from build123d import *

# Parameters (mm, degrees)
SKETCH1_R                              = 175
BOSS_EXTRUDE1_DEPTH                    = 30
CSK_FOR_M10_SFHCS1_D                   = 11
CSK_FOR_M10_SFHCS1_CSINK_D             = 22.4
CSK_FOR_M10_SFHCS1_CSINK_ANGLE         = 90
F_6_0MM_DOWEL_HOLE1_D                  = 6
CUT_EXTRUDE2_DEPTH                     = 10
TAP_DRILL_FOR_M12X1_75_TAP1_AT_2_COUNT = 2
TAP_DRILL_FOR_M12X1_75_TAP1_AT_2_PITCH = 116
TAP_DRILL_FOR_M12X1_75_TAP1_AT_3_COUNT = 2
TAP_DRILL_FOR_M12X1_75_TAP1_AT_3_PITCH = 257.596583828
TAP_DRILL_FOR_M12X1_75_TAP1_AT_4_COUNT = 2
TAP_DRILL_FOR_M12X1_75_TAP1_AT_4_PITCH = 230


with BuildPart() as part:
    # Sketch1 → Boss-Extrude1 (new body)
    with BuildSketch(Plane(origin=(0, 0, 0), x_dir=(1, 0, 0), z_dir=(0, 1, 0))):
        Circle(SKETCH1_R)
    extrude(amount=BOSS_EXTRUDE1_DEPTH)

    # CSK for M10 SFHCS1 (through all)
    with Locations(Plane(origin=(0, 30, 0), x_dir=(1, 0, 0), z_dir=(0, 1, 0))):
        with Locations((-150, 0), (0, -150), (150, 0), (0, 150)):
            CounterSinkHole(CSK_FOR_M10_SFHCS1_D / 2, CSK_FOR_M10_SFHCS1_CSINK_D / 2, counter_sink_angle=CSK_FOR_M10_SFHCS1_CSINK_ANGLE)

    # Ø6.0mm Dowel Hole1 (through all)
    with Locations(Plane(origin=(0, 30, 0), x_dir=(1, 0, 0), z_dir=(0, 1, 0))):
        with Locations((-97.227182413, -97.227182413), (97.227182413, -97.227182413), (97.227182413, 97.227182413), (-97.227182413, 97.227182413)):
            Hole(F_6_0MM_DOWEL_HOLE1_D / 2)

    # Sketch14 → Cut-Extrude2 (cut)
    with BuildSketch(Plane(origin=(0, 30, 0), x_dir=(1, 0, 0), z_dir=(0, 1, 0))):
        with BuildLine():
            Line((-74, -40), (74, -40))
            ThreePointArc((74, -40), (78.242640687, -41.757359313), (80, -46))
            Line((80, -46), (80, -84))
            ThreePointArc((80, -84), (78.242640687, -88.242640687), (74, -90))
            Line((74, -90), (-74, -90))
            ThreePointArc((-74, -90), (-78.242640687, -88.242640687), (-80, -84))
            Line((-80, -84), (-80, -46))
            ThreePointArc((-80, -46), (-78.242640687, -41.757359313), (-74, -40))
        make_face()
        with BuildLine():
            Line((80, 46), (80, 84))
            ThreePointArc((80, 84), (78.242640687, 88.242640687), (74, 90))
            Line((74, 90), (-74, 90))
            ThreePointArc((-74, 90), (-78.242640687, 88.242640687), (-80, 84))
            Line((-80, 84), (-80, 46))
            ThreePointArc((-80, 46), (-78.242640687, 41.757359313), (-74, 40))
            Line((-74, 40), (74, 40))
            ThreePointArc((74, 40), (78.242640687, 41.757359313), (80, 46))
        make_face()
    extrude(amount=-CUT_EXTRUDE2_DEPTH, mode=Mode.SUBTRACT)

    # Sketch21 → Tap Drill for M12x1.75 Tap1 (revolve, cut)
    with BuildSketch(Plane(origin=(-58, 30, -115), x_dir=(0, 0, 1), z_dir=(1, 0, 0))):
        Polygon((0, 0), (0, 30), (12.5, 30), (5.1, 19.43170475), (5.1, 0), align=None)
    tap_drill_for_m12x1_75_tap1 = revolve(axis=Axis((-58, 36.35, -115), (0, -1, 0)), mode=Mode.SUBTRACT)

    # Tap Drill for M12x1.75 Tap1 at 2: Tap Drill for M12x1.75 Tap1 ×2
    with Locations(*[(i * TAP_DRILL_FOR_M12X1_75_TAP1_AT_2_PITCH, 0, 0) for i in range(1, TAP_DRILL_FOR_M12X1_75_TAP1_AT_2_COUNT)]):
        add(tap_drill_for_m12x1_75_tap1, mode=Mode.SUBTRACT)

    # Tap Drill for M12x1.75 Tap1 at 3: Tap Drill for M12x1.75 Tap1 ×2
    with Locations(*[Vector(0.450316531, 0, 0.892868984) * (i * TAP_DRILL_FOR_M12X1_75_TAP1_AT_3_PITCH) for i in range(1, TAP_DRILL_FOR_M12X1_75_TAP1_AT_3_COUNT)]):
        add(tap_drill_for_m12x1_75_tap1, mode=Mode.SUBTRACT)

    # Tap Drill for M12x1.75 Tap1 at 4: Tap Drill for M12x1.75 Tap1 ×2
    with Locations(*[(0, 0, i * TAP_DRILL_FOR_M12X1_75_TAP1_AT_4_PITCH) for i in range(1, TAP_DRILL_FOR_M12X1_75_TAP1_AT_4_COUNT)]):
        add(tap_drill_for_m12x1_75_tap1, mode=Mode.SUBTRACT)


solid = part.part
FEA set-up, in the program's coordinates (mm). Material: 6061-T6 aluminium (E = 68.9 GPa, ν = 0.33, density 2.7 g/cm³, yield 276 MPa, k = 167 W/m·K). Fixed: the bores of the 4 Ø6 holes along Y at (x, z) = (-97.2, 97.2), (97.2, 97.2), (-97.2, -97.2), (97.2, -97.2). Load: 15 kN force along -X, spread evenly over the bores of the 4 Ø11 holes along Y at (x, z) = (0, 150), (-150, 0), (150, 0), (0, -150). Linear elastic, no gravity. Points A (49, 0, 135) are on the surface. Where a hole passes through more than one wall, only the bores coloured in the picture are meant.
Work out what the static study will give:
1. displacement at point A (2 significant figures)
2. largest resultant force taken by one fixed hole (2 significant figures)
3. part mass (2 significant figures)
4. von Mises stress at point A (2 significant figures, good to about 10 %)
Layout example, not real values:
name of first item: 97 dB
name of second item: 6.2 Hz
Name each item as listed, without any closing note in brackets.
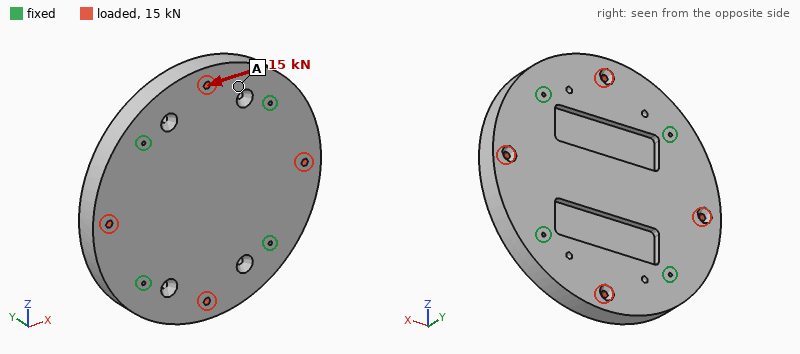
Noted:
displacement at point A: 2.1 µm
largest resultant force taken by one fixed hole: 3.9 kN
part mass: 7.3 kg
von Mises stress at point A: 1.6 MPa
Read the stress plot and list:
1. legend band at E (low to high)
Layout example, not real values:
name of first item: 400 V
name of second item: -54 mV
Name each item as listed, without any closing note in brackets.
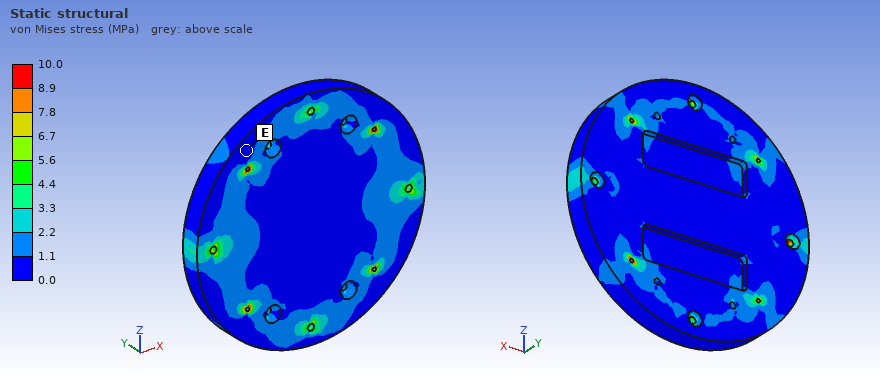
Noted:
legend band at E: 0.0 to 1.1 MPa
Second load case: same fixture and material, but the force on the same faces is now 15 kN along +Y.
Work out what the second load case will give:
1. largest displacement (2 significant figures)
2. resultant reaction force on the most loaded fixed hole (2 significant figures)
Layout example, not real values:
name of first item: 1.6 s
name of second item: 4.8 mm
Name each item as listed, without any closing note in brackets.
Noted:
largest displacement: 44 µm
resultant reaction force on the most loaded fixed hole: 3.8 kN
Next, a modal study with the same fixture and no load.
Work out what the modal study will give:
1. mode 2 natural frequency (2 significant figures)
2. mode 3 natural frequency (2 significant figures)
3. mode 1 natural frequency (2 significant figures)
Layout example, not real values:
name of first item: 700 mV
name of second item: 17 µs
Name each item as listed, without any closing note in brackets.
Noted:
mode 2 natural frequency: 2100 Hz
mode 3 natural frequency: 2200 Hz
mode 1 natural frequency: 1900 Hz
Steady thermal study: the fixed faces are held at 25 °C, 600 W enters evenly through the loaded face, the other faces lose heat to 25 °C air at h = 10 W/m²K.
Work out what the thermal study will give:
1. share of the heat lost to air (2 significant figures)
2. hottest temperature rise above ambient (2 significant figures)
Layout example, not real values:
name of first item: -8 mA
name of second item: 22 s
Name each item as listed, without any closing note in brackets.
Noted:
share of the heat lost to air: 6.3 %
hottest temperature rise above ambient: 34 K
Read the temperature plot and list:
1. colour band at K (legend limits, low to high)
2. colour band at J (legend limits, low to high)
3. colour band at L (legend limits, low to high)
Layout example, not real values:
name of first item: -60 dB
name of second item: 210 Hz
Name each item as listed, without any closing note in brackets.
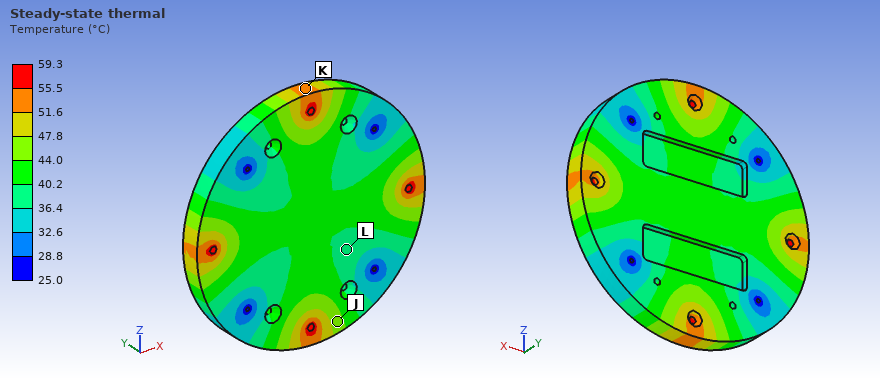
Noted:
colour band at K: 51.6 to 55.5 °C
colour band at J: 44.0 to 47.8 °C
colour band at L: 36.4 to 40.2 °C
